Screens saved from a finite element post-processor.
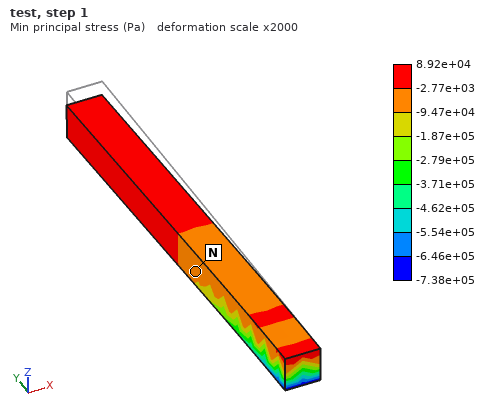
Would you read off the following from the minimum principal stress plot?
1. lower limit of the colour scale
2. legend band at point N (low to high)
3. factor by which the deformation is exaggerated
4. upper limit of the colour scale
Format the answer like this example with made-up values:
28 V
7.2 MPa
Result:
-7.38e+05 Pa
-9.47e+04 to -2.77e+03 Pa
2000
8.92e+04 Pa
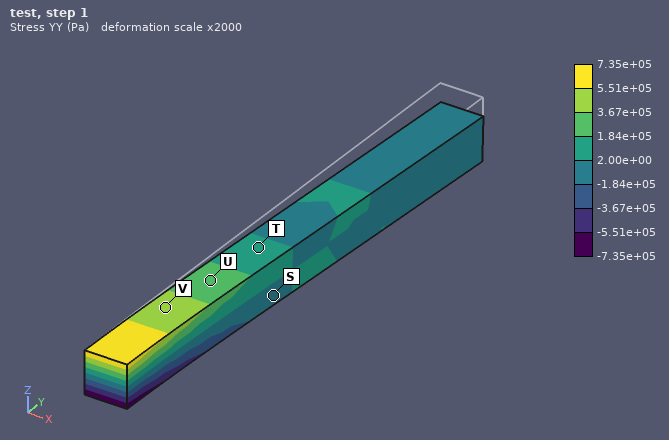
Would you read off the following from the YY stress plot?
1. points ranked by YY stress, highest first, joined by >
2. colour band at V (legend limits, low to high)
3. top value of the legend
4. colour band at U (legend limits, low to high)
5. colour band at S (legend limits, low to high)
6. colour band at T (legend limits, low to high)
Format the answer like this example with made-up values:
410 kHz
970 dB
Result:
V > U > T > S
3.67e+05 to 5.51e+05 Pa
7.35e+05 Pa
1.84e+05 to 3.67e+05 Pa
-1.84e+05 to 2.00e+00 Pa
2.00e+00 to 1.84e+05 Pa
